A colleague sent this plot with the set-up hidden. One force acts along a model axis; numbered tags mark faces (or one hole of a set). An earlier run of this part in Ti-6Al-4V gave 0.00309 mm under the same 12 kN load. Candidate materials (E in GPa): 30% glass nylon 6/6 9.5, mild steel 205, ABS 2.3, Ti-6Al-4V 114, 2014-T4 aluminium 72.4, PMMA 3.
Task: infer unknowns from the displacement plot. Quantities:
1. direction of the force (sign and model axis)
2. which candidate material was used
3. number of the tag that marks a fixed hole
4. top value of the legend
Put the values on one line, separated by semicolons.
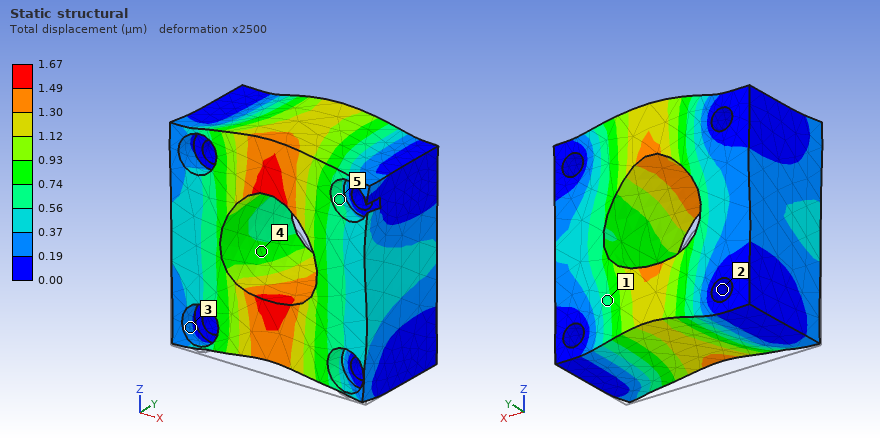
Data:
+Z; mild steel; 2; 1.67 µm
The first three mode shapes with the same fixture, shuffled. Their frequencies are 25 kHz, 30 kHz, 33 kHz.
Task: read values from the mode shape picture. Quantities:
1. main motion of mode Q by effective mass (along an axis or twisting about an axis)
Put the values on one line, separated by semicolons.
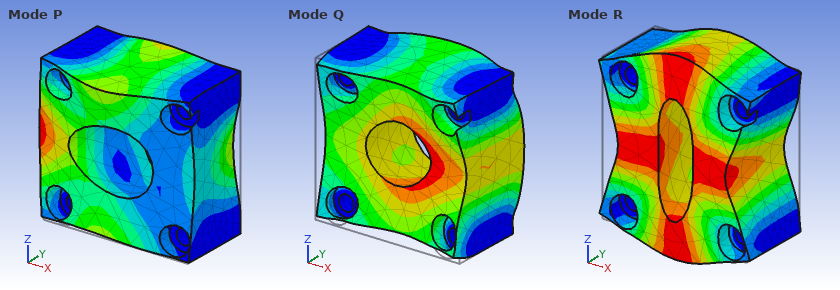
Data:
along Y
